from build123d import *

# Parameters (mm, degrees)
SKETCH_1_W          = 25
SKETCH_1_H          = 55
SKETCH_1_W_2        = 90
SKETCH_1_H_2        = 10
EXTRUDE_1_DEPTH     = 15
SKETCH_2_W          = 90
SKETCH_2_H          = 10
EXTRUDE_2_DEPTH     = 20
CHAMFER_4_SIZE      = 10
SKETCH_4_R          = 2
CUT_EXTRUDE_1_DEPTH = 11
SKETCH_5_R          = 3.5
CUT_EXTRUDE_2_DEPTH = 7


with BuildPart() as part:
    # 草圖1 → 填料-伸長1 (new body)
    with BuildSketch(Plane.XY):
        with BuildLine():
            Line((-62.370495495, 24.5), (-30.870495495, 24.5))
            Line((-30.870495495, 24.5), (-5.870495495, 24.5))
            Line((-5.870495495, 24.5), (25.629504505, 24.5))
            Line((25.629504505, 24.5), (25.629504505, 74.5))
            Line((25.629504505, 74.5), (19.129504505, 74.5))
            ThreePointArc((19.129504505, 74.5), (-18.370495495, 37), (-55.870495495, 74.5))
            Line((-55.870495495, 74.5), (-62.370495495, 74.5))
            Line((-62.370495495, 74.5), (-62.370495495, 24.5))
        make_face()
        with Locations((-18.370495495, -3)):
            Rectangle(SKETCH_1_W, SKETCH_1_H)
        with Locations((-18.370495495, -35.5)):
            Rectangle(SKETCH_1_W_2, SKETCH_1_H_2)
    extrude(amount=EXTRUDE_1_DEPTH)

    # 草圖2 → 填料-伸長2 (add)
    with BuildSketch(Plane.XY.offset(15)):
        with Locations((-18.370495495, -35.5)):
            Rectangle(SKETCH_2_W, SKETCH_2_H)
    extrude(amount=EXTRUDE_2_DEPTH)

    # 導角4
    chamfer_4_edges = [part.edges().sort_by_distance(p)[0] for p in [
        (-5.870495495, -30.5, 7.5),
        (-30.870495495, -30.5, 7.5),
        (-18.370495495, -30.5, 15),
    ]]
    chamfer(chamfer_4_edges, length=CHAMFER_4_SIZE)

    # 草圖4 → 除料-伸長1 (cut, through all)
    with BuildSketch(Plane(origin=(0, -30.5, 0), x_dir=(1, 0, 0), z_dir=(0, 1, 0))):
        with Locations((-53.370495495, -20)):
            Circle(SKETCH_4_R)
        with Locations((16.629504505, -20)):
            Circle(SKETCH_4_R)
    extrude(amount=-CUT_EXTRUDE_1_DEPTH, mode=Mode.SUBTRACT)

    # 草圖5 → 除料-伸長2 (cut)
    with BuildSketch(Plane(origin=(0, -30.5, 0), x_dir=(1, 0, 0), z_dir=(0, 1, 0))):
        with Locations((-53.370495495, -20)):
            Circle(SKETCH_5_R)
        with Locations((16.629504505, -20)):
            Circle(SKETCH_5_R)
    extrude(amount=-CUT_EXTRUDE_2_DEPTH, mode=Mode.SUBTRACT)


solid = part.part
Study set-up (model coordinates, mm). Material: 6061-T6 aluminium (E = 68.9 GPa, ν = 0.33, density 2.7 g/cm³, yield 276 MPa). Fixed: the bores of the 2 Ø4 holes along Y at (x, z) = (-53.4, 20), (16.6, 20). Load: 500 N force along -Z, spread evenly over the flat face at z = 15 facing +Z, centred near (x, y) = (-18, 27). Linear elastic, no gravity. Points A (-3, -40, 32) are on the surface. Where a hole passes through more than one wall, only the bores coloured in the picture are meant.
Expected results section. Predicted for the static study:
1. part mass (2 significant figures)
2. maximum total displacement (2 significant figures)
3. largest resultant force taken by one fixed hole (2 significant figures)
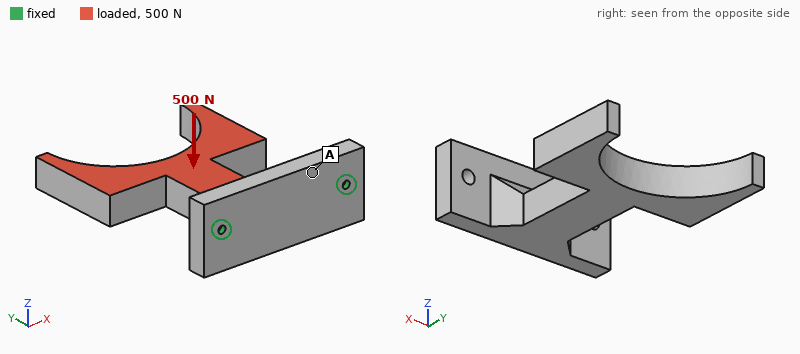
240 g
1.0 mm
270 N
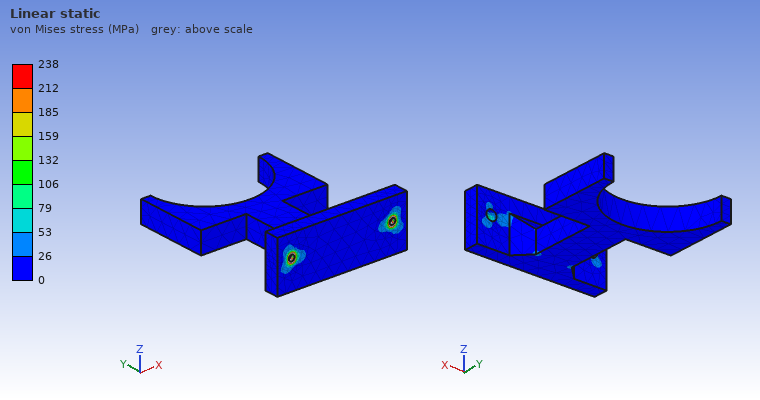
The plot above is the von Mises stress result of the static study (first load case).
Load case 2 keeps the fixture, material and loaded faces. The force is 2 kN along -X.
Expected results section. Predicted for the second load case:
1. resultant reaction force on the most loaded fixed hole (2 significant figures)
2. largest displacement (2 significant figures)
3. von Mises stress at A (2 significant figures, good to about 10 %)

2.2 kN
0.43 mm
21 MPa
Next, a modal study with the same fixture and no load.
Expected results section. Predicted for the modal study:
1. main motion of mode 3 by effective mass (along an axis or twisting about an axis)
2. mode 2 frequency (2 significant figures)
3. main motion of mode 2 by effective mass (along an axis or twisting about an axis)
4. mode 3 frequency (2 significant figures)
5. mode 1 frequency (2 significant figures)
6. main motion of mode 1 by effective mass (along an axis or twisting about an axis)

twisting about Y
1200 Hz
along X
1400 Hz
380 Hz
along Z
